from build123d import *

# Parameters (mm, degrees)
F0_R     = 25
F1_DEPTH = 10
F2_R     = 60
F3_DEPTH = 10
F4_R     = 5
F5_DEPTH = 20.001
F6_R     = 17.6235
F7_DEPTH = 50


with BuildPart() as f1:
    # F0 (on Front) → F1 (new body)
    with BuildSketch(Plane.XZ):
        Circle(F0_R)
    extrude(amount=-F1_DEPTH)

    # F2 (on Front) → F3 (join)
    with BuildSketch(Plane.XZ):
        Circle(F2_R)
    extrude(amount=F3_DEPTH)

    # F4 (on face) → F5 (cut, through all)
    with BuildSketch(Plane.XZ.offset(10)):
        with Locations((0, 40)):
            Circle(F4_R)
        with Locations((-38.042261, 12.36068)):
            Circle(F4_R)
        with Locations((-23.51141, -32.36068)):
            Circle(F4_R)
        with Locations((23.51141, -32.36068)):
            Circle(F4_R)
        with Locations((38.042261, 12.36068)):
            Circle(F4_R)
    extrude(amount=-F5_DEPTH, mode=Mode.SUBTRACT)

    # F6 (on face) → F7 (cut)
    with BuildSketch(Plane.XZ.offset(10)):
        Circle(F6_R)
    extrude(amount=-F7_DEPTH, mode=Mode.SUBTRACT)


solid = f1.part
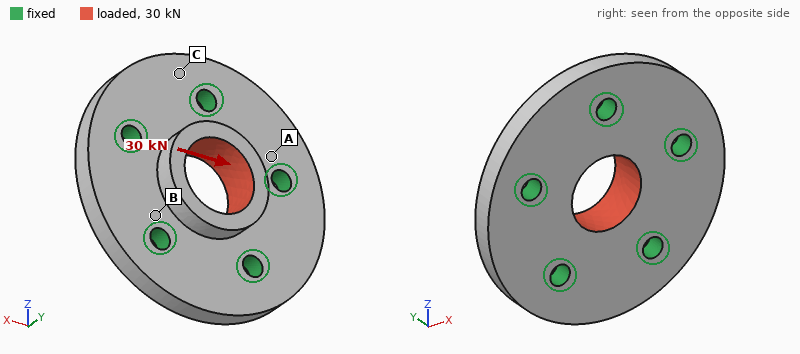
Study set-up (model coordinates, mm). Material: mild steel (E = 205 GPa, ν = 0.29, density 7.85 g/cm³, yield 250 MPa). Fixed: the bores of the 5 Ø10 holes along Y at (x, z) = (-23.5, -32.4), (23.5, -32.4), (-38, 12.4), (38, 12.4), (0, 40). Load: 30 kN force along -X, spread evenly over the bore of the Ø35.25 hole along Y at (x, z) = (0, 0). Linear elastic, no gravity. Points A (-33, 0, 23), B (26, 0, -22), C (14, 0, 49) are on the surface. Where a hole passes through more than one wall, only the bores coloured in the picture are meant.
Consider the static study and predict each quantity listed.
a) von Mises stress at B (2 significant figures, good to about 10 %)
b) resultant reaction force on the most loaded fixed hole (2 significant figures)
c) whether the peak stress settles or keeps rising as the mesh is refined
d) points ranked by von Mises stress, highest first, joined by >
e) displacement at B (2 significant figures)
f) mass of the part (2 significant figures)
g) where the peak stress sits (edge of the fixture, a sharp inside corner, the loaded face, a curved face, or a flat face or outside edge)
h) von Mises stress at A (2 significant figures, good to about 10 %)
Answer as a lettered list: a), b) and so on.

a) 18 MPa
b) 7.8 kN
c) keeps rising
d) B > A > C
e) 1.4 µm
f) 860 g
g) edge of the fixture
h) 9.5 MPa
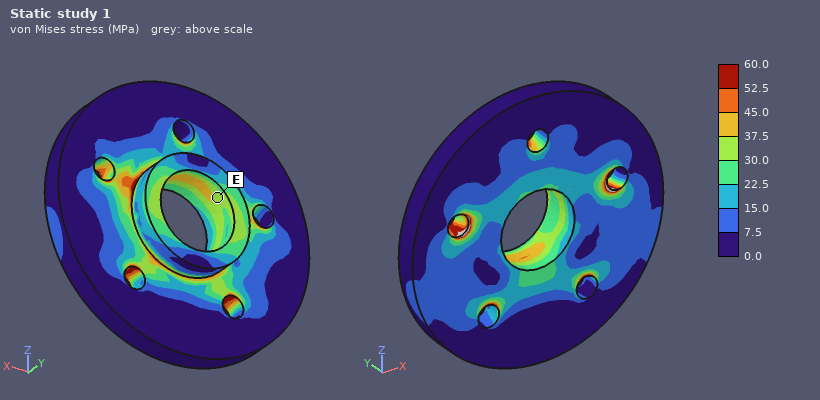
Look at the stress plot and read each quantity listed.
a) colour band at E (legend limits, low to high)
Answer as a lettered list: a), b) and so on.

a) 30.0 to 37.5 MPa
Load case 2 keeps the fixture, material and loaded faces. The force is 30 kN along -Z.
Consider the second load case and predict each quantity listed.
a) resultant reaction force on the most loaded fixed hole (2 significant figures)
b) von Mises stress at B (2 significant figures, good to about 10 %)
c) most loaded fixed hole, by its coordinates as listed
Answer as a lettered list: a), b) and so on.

a) 8.1 kN
b) 23 MPa
c) (0, 40)
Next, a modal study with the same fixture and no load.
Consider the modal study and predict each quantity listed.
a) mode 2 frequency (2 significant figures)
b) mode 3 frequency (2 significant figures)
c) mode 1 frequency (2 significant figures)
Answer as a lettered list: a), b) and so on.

a) 11 kHz
b) 12 kHz
c) 11 kHz
